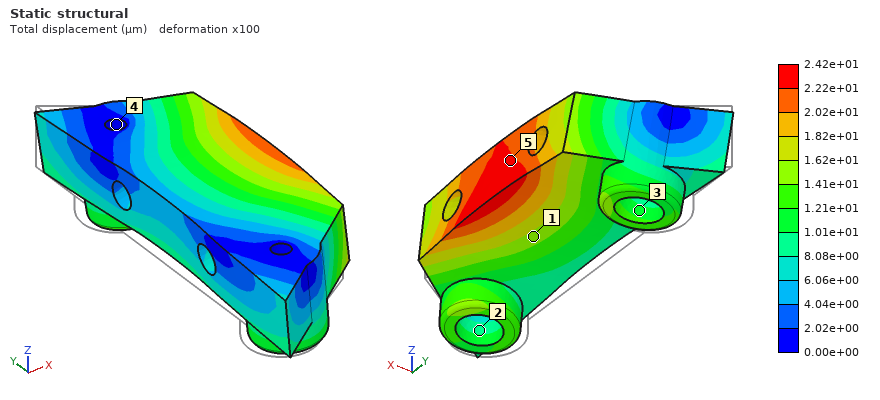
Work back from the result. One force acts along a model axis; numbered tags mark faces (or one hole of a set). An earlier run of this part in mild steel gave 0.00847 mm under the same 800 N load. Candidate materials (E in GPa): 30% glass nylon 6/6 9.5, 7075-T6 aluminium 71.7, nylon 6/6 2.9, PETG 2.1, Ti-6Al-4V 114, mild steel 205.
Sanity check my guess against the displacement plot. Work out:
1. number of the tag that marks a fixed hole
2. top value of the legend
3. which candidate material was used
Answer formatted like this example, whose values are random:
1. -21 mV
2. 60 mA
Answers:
1. 4
2. 2.42e+01 µm
3. 7075-T6 aluminium
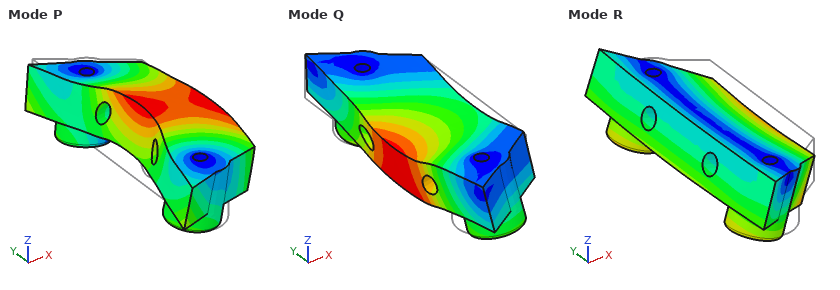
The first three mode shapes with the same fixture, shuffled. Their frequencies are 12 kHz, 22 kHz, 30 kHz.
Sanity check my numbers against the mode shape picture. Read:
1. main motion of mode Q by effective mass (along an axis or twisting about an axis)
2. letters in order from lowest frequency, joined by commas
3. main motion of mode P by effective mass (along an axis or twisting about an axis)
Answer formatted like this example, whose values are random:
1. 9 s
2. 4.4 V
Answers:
1. along Z
2. R, Q, P
3. along X
